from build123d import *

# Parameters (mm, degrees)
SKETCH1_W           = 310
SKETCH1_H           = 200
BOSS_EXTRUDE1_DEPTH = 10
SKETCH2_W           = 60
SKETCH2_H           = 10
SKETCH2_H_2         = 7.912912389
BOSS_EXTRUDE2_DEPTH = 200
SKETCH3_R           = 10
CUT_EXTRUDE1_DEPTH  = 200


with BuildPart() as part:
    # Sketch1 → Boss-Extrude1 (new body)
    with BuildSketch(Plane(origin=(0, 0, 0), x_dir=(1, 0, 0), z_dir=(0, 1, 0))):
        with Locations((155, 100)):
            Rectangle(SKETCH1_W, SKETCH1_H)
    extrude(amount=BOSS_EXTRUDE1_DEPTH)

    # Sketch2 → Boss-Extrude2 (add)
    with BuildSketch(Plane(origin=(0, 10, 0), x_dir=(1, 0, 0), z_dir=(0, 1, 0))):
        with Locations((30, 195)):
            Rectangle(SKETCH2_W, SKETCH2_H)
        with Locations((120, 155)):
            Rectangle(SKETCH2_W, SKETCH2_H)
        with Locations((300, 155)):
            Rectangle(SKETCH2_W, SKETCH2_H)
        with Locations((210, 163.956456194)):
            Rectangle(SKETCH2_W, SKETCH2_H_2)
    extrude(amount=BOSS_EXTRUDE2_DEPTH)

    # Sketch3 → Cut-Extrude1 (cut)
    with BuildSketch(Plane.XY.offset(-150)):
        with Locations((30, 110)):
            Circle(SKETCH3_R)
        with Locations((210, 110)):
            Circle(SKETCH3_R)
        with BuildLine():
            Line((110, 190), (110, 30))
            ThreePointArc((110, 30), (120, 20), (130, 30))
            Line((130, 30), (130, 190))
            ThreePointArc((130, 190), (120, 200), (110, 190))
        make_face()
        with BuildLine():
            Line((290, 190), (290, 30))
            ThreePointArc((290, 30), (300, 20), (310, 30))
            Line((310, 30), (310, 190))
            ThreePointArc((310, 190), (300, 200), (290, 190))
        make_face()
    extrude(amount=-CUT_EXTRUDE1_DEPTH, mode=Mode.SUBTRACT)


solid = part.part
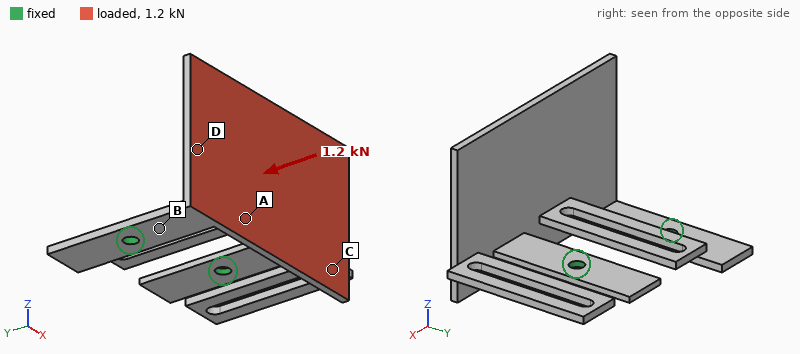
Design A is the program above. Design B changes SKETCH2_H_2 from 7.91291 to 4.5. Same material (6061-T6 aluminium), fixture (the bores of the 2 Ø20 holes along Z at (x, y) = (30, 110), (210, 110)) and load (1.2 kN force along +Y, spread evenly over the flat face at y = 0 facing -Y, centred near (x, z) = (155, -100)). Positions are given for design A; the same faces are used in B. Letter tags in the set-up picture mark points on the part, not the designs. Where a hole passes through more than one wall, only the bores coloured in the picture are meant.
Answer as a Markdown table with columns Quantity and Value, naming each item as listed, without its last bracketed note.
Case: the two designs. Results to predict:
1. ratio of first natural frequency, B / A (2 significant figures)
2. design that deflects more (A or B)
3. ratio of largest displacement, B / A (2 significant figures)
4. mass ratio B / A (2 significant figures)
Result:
| Quantity | Value |
|---|---|
| ratio of first natural frequency, B / A | 0.83 |
| design that deflects more | B |
| ratio of largest displacement, B / A | 1.4 |
| mass ratio B / A | 0.96 |
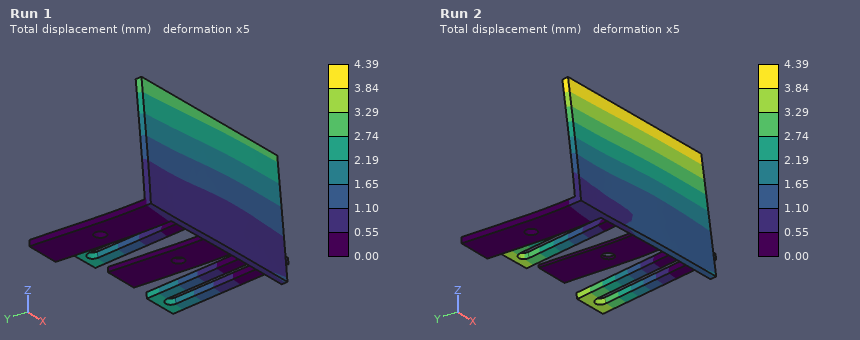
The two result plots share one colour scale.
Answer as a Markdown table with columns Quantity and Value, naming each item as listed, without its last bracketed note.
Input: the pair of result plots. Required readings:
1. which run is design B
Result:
| Quantity | Value |
|---|---|
| which run is design B | Run 2 |
